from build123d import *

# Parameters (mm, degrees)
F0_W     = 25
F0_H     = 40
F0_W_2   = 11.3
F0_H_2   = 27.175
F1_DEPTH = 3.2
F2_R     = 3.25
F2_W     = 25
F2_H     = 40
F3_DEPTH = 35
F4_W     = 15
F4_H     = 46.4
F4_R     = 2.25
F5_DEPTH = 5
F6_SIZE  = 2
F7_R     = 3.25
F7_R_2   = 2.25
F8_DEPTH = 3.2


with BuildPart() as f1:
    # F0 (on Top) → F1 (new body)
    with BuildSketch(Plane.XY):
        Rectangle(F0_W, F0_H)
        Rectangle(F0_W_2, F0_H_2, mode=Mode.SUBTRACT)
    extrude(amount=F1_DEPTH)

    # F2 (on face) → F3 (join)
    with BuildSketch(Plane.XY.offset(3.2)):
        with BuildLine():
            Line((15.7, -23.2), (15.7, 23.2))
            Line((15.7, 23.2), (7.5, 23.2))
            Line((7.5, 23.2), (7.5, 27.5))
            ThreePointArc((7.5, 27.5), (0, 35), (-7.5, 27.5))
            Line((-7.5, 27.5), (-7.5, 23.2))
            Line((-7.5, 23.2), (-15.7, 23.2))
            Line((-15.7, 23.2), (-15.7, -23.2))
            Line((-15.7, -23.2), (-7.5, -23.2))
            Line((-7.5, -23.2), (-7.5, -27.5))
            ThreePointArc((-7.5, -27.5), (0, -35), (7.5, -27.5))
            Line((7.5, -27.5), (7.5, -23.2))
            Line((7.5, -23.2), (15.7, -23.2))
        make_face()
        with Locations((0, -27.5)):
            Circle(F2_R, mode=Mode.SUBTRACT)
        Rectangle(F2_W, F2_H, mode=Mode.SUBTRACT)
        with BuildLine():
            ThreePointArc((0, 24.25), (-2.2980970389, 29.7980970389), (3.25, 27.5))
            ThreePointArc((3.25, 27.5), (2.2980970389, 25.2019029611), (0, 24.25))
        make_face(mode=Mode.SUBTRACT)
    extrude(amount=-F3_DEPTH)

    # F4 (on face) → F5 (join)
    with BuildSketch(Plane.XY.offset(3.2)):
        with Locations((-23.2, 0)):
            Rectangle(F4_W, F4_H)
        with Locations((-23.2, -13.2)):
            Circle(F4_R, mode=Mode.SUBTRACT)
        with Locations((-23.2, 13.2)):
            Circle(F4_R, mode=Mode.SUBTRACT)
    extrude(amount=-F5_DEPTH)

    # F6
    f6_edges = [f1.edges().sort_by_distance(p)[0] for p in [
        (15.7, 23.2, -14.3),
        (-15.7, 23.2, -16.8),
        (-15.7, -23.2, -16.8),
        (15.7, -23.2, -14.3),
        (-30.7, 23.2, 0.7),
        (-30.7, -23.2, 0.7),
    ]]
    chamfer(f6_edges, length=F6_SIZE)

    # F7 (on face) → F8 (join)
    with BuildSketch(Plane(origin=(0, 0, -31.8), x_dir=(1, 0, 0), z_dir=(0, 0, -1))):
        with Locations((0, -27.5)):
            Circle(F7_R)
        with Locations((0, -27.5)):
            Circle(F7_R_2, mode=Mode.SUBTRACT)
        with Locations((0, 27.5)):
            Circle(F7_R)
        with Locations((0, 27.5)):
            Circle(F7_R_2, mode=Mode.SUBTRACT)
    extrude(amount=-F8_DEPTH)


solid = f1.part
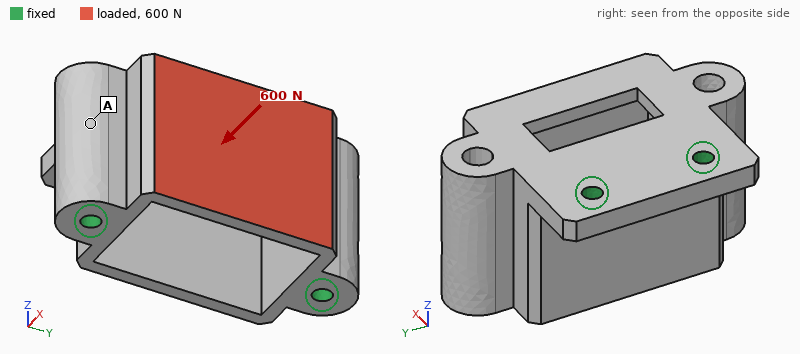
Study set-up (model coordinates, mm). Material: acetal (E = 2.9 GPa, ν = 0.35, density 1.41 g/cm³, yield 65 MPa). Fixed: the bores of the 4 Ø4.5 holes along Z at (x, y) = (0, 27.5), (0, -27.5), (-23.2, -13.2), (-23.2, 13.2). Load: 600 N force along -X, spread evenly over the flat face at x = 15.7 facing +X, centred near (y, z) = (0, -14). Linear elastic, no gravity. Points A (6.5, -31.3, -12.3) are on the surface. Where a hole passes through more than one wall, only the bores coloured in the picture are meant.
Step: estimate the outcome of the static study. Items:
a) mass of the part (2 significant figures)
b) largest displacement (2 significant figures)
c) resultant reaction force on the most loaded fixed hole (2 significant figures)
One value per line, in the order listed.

42 g
0.65 mm
190 N
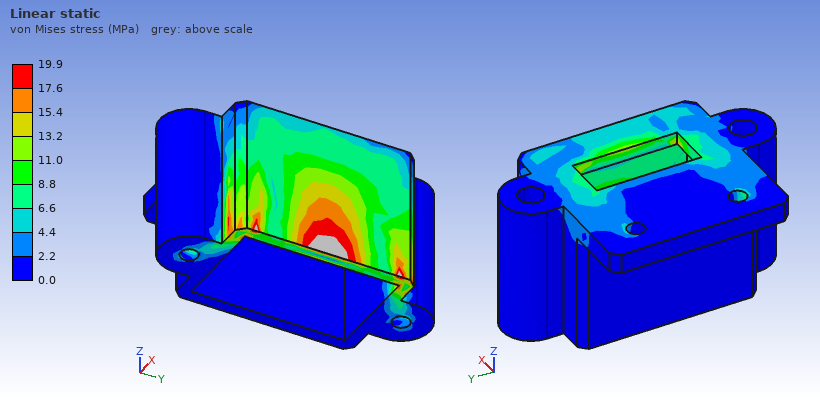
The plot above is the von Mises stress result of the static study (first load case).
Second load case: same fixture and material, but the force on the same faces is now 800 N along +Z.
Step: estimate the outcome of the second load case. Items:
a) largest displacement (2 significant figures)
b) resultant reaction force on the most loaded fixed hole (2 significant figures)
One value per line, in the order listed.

0.20 mm
440 N
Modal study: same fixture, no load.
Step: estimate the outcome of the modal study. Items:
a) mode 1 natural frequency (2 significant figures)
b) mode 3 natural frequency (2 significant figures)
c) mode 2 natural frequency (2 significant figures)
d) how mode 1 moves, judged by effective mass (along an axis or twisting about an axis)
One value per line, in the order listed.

2100 Hz
2600 Hz
2400 Hz
along Y
